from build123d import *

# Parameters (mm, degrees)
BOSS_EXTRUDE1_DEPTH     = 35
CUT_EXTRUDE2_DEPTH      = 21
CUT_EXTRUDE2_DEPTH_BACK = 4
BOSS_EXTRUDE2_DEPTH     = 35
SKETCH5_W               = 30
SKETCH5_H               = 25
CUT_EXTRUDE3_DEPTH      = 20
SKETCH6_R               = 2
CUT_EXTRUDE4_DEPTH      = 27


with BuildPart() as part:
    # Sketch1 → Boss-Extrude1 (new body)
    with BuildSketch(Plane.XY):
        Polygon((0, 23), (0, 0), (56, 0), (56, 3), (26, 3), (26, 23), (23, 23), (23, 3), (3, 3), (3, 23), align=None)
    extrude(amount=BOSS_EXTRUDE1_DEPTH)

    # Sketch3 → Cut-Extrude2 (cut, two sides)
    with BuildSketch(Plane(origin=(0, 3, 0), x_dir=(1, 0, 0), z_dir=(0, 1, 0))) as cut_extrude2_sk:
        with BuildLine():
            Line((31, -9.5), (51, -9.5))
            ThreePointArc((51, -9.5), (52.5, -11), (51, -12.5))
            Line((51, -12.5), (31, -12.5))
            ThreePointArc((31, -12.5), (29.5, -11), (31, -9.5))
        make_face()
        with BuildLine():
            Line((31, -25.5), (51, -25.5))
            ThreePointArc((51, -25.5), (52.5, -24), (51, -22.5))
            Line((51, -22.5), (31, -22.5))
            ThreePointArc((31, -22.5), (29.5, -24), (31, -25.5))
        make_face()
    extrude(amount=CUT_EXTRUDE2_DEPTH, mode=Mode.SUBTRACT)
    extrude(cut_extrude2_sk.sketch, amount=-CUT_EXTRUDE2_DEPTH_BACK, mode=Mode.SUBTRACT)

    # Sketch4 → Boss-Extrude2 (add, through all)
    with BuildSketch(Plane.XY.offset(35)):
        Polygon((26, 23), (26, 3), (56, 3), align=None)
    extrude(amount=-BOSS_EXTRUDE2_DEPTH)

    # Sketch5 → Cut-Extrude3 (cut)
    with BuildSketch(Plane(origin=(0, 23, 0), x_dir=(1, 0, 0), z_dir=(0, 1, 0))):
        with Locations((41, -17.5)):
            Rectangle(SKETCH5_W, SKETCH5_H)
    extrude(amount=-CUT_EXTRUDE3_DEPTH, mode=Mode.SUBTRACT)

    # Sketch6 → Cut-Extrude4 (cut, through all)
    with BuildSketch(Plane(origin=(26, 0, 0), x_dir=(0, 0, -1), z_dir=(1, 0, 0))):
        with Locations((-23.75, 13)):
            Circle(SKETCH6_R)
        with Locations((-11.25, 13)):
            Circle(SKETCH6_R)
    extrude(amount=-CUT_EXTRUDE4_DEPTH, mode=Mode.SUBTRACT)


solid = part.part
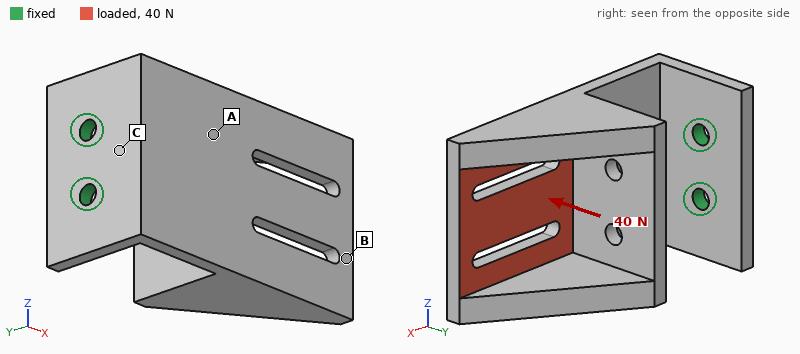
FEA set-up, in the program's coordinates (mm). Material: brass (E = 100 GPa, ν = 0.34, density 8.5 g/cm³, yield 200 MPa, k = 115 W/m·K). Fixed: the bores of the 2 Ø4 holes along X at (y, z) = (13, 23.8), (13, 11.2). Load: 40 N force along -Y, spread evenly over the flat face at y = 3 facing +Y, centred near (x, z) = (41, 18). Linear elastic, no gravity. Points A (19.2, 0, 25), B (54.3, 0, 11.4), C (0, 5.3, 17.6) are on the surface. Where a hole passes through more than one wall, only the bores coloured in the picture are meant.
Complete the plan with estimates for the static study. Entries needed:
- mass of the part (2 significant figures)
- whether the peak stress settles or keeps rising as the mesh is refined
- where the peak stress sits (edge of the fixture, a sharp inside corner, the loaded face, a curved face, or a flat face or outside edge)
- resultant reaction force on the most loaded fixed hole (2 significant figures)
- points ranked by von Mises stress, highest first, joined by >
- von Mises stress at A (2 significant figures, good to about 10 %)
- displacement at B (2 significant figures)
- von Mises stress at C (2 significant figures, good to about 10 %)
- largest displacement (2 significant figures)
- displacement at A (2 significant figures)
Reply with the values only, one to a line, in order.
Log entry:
110 g
keeps rising
edge of the fixture
22 N
C > A > B
15 MPa
0.23 mm
28 MPa
0.24 mm
0.061 mm
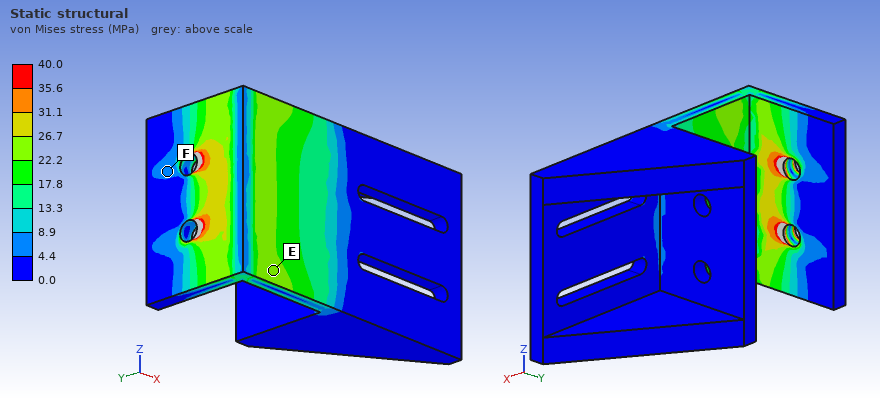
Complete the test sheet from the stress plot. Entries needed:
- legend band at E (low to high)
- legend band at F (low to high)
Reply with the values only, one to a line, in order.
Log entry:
22.2 to 26.7 MPa
4.4 to 8.9 MPa
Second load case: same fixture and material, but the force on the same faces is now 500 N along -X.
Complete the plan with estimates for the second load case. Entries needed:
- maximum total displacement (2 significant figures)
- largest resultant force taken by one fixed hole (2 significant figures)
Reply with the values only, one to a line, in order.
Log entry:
75 µm
250 N
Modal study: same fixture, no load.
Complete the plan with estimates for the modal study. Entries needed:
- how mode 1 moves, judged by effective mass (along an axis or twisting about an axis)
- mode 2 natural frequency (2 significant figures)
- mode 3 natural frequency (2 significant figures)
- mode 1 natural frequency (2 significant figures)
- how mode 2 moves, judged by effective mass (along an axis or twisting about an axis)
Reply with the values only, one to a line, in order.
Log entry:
along Y
730 Hz
1400 Hz
340 Hz
along Z
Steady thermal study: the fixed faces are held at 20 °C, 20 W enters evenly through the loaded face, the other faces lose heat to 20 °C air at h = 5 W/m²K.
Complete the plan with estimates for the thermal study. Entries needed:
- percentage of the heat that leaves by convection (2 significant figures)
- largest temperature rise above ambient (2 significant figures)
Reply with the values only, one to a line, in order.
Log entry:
8.4 %
76 K
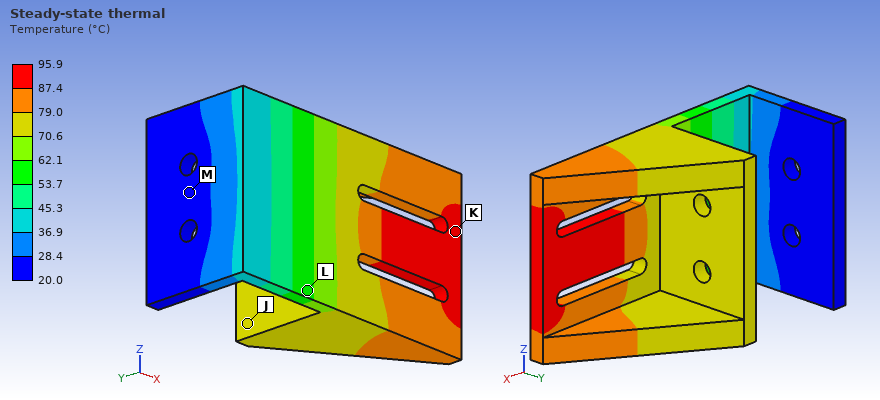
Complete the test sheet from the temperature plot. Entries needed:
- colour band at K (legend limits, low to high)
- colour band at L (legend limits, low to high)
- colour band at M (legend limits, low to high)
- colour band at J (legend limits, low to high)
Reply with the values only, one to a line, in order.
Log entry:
87.4 to 95.9 °C
53.7 to 62.1 °C
20.0 to 28.4 °C
70.6 to 79.0 °C
